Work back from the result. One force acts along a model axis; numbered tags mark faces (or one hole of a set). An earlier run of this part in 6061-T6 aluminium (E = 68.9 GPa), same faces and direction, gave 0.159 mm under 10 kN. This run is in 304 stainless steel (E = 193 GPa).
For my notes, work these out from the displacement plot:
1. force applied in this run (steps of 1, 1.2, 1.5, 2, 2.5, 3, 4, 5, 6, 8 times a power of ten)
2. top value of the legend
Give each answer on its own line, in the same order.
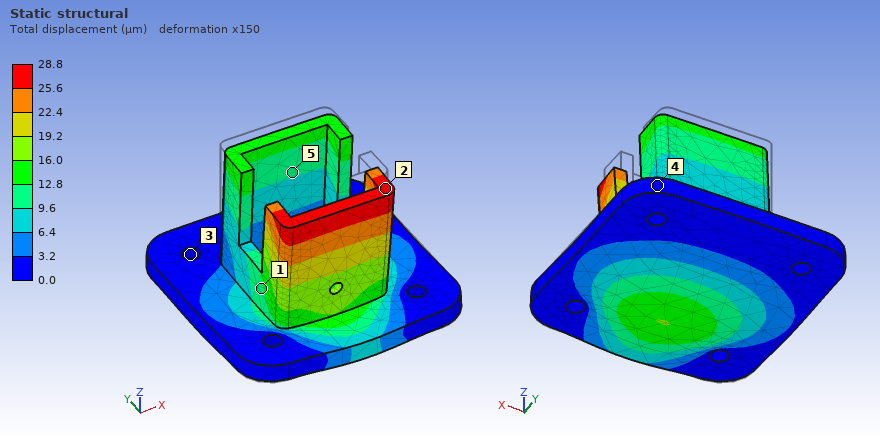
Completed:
5 kN
28.8 µm
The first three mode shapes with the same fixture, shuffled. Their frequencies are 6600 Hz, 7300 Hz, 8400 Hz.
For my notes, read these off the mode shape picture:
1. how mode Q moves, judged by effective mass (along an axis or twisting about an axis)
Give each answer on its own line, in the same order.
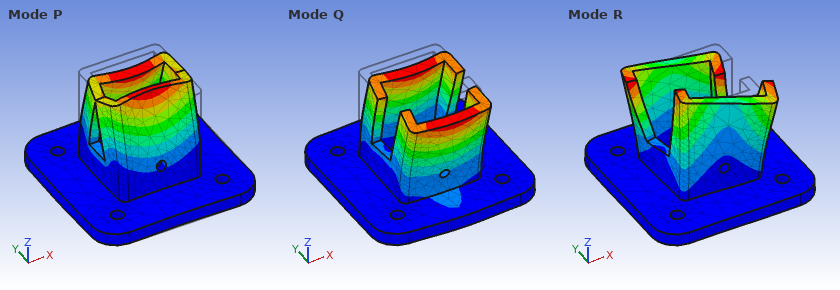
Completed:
along Y
